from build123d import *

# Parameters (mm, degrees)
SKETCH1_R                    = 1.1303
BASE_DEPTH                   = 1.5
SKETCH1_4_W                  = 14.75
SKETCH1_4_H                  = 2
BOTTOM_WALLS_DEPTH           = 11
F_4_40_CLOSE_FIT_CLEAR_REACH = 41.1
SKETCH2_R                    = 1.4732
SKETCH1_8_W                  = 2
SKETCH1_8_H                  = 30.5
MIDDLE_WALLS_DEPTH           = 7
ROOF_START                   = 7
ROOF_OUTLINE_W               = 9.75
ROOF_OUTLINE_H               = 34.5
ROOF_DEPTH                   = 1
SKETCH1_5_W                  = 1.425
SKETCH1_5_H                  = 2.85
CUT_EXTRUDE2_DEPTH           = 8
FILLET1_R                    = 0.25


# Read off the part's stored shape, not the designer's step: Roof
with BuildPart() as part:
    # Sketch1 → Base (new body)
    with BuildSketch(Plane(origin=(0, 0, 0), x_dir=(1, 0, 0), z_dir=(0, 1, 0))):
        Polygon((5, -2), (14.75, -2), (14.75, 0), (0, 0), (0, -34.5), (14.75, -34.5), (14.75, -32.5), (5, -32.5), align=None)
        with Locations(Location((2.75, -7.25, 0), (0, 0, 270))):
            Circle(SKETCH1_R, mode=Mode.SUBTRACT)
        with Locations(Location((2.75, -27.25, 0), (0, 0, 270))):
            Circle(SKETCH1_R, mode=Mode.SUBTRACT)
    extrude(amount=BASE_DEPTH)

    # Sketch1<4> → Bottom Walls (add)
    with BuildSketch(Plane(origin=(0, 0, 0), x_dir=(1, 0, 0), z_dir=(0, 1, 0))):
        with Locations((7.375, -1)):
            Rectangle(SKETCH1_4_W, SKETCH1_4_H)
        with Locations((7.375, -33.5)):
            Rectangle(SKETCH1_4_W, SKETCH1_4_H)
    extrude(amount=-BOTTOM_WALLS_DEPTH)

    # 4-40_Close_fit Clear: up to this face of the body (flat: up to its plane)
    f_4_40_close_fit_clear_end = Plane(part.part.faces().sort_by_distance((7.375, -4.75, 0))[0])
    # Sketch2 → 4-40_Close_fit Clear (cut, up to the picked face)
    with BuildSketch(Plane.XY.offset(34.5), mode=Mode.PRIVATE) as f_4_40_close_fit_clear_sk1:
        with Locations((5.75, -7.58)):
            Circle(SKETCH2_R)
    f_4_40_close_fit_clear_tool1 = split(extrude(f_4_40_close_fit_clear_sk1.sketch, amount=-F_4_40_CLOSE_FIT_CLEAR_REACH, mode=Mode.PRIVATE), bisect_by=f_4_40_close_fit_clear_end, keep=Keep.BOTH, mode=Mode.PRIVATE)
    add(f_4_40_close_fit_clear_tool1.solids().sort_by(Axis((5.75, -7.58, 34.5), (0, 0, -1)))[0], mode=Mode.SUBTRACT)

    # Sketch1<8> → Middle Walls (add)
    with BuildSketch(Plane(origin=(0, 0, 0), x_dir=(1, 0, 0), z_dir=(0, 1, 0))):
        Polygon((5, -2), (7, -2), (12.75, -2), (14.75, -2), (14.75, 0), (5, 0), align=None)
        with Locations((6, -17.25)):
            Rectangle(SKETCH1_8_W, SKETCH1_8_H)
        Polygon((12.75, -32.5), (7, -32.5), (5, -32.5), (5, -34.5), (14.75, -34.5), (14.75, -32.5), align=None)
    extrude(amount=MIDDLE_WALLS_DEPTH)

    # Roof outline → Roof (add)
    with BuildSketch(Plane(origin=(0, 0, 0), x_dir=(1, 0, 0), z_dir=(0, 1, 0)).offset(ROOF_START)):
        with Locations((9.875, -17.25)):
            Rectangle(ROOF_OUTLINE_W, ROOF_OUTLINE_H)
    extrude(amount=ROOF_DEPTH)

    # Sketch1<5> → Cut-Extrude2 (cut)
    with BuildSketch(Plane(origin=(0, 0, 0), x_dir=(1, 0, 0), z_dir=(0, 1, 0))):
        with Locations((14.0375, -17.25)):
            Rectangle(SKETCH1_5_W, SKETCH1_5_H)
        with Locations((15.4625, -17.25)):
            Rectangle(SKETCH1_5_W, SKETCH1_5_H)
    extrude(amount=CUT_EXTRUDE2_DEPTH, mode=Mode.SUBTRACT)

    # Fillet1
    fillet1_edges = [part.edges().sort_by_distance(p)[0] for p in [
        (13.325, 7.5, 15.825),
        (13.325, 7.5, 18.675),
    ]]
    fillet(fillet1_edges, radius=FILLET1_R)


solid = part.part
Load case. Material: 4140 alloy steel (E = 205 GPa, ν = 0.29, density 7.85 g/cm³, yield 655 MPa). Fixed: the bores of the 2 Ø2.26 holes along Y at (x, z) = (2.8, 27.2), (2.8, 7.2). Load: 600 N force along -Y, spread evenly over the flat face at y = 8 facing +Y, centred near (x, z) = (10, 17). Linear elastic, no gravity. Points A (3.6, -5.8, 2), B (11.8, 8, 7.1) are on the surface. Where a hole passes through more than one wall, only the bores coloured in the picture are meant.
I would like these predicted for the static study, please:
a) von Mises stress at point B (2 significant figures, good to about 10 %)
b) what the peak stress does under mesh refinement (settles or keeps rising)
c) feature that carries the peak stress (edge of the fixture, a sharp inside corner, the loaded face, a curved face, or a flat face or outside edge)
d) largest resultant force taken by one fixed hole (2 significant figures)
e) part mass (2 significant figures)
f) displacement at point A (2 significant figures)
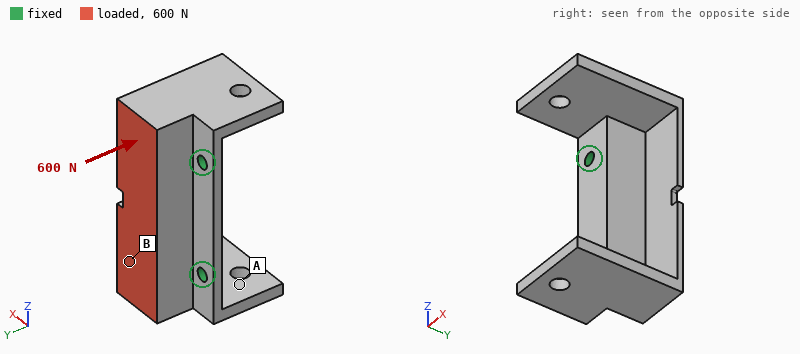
99 MPa
keeps rising
edge of the fixture
300 N
15 g
0.037 mm
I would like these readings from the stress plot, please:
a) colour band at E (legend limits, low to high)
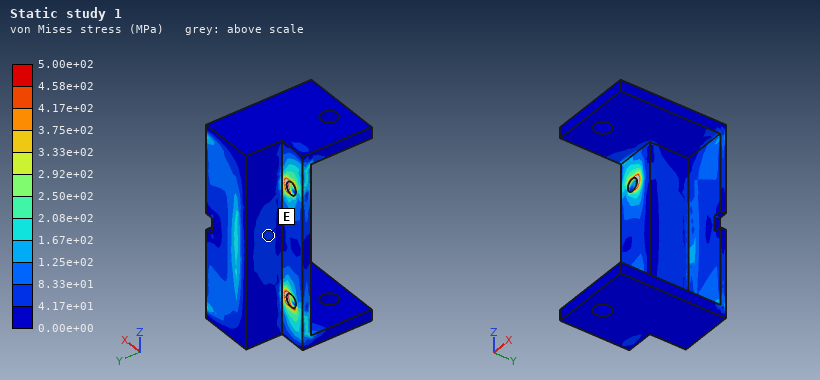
4.17e+01 to 8.33e+01 MPa
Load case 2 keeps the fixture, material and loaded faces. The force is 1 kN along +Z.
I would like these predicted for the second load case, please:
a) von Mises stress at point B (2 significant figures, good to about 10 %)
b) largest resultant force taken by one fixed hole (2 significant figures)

19 MPa
670 N
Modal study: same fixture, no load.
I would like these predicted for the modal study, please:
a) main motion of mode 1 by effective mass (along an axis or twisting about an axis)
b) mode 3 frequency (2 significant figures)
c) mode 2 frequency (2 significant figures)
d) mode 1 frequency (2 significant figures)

along Y
7000 Hz
5000 Hz
4300 Hz
